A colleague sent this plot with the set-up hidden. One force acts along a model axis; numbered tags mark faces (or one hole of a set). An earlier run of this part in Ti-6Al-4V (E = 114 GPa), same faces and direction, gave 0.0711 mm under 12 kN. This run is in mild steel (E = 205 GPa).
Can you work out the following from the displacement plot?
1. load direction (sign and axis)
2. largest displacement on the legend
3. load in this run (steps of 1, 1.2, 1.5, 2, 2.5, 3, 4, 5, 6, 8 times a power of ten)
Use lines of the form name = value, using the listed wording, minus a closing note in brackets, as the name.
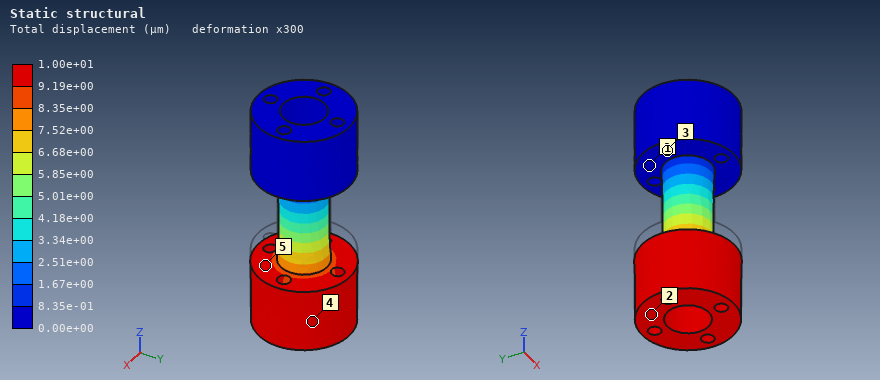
load direction = -Z
largest displacement on the legend = 1.00e+01 µm
load in this run = 3 kN
